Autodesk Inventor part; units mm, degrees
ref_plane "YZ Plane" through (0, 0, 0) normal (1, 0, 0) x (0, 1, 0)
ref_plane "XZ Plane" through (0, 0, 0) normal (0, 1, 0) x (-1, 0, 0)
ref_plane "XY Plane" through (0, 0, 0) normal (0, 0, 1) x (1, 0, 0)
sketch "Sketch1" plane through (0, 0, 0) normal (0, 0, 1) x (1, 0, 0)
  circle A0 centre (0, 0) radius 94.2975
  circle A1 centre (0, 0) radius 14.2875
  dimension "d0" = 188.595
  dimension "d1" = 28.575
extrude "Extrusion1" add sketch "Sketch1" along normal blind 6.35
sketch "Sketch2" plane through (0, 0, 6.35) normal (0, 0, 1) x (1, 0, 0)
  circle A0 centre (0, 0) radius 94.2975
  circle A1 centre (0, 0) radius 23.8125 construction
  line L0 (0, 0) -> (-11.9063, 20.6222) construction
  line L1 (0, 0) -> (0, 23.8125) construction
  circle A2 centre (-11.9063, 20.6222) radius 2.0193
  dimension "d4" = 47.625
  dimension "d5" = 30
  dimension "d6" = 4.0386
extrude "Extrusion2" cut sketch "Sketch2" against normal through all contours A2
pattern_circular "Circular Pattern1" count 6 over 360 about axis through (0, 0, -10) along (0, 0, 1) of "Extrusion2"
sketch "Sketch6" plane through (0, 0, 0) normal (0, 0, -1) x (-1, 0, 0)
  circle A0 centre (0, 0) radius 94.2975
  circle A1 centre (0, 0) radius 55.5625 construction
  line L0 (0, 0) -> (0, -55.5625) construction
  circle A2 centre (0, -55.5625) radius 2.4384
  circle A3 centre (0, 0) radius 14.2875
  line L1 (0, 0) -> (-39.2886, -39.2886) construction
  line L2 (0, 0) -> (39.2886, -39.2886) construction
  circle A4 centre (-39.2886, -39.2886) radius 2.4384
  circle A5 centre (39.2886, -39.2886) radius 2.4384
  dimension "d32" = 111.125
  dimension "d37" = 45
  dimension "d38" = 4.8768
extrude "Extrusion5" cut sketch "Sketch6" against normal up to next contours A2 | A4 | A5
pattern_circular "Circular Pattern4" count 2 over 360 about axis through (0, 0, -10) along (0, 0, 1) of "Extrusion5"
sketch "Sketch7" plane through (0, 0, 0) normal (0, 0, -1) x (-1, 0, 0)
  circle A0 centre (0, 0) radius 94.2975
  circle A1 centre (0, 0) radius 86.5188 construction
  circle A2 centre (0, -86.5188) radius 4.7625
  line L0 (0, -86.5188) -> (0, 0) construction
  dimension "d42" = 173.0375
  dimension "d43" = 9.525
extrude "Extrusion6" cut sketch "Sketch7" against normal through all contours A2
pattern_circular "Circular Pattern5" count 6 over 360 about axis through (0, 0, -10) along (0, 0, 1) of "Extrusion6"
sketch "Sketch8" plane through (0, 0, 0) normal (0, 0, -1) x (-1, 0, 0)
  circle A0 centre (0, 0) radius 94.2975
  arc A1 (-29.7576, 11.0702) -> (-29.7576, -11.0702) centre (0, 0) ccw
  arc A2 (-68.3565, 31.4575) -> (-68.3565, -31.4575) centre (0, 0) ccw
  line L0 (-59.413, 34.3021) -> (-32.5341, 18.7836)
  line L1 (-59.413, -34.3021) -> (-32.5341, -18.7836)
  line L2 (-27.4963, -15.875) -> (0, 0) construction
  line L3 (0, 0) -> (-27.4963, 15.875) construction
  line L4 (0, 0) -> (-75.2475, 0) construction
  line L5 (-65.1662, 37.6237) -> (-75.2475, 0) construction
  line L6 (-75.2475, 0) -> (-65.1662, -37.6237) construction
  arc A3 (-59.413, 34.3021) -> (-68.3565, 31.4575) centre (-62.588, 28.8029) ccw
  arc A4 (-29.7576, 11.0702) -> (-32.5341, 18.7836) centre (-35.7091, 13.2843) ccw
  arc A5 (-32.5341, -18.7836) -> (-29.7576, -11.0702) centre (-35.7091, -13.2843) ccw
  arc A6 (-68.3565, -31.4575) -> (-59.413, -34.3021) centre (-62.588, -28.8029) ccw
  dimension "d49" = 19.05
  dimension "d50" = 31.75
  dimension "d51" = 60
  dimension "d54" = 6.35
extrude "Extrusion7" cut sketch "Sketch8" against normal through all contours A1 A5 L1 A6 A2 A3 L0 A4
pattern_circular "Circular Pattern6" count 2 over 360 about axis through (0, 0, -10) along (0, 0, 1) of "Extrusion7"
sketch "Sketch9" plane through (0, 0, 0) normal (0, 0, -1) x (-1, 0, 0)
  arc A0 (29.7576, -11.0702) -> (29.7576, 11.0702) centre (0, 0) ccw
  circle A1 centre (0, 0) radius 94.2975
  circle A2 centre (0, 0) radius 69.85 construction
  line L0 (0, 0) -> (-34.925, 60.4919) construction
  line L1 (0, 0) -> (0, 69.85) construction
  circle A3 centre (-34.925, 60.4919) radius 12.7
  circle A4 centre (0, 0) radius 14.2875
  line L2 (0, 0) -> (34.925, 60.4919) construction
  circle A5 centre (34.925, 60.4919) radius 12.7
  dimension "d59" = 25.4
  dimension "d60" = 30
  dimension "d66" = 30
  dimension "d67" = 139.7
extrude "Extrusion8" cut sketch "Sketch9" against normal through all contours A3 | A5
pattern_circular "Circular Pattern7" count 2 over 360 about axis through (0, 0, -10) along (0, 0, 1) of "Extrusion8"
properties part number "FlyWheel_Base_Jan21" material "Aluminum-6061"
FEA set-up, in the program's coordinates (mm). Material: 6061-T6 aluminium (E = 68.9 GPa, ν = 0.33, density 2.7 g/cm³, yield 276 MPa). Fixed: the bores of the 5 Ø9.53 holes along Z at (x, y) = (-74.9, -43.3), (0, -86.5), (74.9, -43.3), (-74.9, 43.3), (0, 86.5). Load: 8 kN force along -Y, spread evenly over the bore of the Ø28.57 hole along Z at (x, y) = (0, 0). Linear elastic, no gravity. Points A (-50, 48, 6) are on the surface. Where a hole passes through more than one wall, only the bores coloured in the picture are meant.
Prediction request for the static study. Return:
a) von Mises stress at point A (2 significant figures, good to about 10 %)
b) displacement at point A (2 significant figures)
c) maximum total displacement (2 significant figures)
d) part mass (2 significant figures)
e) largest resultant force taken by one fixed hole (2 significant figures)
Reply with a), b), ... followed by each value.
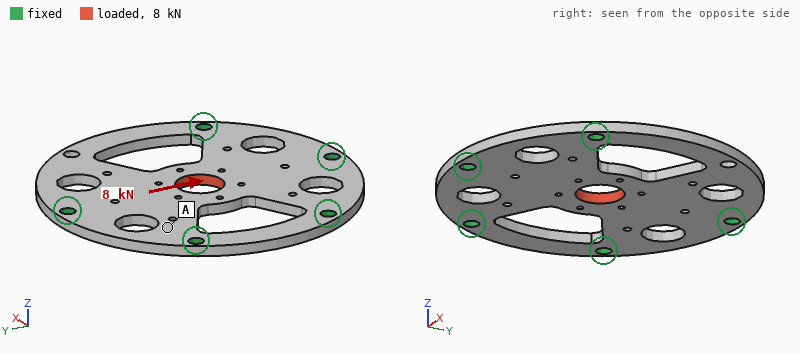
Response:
a) 3.0 MPa
b) 4.6 µm
c) 16 µm
d) 340 g
e) 3.0 kN
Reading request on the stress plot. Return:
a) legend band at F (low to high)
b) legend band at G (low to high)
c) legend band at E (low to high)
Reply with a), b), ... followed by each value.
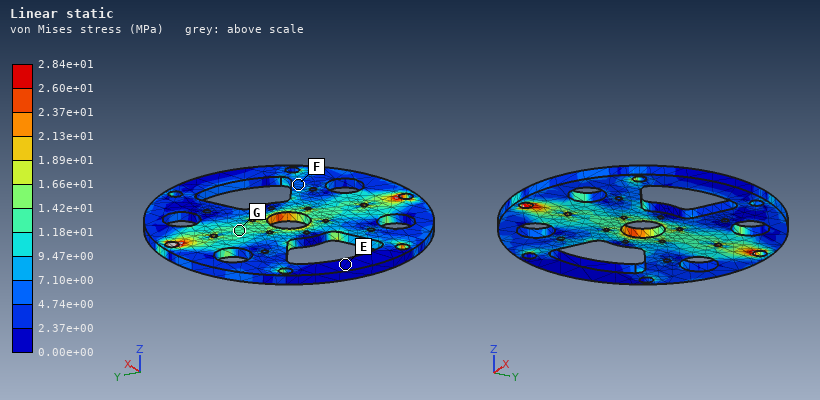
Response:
a) 4.74e+00 to 7.10e+00 MPa
b) 1.18e+01 to 1.42e+01 MPa
c) 0.00e+00 to 2.37e+00 MPa
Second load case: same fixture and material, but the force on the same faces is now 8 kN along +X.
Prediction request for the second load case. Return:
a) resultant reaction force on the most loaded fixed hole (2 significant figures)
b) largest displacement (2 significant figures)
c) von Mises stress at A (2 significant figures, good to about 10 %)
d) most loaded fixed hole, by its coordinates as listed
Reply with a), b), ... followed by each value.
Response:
a) 2.5 kN
b) 31 µm
c) 12 MPa
d) (-74.9, 43.3)
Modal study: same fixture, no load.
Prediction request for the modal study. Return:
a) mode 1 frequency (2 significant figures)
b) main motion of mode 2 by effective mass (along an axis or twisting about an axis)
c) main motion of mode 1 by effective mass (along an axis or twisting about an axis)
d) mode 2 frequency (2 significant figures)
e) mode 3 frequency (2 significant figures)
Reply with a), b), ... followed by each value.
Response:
a) 1100 Hz
b) along Z
c) along Z
d) 1600 Hz
e) 2900 Hz
